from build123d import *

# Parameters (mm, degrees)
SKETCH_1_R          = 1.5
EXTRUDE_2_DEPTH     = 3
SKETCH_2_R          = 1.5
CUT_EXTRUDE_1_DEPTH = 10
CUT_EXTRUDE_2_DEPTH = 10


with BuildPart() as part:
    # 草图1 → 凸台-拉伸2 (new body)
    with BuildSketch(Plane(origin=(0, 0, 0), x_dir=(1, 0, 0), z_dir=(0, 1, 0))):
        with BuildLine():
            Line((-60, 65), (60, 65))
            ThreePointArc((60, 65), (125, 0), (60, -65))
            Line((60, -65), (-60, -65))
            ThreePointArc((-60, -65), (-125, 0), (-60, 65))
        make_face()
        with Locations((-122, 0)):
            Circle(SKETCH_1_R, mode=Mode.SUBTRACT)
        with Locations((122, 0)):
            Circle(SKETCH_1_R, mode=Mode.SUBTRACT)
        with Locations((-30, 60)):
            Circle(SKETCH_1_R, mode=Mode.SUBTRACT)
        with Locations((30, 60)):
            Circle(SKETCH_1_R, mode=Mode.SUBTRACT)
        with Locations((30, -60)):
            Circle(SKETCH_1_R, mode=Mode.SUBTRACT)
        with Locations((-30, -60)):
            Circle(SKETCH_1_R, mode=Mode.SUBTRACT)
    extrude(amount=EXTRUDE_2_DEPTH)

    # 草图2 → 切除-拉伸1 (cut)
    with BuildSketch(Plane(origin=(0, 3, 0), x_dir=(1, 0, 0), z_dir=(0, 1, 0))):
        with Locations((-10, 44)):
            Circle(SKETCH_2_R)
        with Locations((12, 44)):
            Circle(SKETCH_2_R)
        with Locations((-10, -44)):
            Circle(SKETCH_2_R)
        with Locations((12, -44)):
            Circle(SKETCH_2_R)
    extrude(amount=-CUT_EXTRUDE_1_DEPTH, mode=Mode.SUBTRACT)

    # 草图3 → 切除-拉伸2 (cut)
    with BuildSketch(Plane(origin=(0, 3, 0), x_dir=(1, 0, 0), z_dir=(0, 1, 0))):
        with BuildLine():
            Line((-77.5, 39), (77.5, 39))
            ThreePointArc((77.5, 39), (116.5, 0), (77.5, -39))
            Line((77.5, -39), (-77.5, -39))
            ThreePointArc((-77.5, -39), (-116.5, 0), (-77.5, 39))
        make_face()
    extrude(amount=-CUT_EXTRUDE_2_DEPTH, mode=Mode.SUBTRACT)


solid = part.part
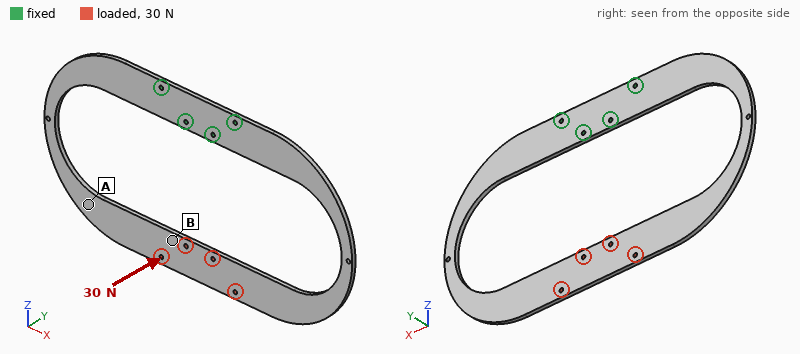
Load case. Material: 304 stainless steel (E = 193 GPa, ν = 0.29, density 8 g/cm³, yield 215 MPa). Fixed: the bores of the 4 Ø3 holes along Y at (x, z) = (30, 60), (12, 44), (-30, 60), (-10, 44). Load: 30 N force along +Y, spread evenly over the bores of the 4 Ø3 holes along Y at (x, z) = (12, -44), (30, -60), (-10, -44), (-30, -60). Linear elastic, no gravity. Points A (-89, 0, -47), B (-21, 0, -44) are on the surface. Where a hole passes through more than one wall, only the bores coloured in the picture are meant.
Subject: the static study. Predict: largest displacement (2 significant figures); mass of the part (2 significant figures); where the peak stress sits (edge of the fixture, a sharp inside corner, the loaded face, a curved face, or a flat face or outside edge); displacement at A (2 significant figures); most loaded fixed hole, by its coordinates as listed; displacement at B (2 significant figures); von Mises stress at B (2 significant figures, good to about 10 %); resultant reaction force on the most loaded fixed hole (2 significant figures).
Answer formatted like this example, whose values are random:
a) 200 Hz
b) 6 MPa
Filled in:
a) 2.7 mm
b) 290 g
c) a curved face
d) 2.0 mm
e) (-30, 60)
f) 2.2 mm
g) 23 MPa
h) 16 N
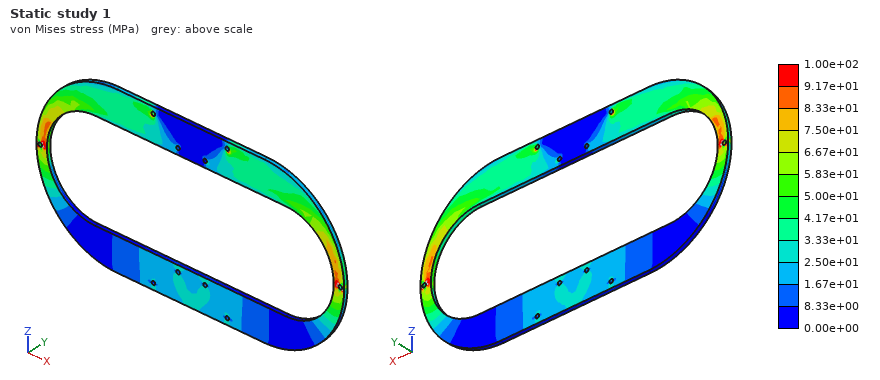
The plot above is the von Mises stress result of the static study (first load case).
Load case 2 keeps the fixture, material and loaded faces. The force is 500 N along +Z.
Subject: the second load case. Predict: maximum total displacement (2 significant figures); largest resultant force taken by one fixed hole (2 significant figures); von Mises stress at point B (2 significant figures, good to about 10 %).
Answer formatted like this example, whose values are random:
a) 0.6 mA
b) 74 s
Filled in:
a) 0.24 mm
b) 1.1 kN
c) 33 MPa
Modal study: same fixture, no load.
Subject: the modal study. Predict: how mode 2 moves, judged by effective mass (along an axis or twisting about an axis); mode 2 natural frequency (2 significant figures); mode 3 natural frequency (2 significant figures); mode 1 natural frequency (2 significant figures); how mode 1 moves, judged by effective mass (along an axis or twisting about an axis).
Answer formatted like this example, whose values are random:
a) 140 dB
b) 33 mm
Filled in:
a) twisting about Z
b) 120 Hz
c) 250 Hz
d) 52 Hz
e) along Y
